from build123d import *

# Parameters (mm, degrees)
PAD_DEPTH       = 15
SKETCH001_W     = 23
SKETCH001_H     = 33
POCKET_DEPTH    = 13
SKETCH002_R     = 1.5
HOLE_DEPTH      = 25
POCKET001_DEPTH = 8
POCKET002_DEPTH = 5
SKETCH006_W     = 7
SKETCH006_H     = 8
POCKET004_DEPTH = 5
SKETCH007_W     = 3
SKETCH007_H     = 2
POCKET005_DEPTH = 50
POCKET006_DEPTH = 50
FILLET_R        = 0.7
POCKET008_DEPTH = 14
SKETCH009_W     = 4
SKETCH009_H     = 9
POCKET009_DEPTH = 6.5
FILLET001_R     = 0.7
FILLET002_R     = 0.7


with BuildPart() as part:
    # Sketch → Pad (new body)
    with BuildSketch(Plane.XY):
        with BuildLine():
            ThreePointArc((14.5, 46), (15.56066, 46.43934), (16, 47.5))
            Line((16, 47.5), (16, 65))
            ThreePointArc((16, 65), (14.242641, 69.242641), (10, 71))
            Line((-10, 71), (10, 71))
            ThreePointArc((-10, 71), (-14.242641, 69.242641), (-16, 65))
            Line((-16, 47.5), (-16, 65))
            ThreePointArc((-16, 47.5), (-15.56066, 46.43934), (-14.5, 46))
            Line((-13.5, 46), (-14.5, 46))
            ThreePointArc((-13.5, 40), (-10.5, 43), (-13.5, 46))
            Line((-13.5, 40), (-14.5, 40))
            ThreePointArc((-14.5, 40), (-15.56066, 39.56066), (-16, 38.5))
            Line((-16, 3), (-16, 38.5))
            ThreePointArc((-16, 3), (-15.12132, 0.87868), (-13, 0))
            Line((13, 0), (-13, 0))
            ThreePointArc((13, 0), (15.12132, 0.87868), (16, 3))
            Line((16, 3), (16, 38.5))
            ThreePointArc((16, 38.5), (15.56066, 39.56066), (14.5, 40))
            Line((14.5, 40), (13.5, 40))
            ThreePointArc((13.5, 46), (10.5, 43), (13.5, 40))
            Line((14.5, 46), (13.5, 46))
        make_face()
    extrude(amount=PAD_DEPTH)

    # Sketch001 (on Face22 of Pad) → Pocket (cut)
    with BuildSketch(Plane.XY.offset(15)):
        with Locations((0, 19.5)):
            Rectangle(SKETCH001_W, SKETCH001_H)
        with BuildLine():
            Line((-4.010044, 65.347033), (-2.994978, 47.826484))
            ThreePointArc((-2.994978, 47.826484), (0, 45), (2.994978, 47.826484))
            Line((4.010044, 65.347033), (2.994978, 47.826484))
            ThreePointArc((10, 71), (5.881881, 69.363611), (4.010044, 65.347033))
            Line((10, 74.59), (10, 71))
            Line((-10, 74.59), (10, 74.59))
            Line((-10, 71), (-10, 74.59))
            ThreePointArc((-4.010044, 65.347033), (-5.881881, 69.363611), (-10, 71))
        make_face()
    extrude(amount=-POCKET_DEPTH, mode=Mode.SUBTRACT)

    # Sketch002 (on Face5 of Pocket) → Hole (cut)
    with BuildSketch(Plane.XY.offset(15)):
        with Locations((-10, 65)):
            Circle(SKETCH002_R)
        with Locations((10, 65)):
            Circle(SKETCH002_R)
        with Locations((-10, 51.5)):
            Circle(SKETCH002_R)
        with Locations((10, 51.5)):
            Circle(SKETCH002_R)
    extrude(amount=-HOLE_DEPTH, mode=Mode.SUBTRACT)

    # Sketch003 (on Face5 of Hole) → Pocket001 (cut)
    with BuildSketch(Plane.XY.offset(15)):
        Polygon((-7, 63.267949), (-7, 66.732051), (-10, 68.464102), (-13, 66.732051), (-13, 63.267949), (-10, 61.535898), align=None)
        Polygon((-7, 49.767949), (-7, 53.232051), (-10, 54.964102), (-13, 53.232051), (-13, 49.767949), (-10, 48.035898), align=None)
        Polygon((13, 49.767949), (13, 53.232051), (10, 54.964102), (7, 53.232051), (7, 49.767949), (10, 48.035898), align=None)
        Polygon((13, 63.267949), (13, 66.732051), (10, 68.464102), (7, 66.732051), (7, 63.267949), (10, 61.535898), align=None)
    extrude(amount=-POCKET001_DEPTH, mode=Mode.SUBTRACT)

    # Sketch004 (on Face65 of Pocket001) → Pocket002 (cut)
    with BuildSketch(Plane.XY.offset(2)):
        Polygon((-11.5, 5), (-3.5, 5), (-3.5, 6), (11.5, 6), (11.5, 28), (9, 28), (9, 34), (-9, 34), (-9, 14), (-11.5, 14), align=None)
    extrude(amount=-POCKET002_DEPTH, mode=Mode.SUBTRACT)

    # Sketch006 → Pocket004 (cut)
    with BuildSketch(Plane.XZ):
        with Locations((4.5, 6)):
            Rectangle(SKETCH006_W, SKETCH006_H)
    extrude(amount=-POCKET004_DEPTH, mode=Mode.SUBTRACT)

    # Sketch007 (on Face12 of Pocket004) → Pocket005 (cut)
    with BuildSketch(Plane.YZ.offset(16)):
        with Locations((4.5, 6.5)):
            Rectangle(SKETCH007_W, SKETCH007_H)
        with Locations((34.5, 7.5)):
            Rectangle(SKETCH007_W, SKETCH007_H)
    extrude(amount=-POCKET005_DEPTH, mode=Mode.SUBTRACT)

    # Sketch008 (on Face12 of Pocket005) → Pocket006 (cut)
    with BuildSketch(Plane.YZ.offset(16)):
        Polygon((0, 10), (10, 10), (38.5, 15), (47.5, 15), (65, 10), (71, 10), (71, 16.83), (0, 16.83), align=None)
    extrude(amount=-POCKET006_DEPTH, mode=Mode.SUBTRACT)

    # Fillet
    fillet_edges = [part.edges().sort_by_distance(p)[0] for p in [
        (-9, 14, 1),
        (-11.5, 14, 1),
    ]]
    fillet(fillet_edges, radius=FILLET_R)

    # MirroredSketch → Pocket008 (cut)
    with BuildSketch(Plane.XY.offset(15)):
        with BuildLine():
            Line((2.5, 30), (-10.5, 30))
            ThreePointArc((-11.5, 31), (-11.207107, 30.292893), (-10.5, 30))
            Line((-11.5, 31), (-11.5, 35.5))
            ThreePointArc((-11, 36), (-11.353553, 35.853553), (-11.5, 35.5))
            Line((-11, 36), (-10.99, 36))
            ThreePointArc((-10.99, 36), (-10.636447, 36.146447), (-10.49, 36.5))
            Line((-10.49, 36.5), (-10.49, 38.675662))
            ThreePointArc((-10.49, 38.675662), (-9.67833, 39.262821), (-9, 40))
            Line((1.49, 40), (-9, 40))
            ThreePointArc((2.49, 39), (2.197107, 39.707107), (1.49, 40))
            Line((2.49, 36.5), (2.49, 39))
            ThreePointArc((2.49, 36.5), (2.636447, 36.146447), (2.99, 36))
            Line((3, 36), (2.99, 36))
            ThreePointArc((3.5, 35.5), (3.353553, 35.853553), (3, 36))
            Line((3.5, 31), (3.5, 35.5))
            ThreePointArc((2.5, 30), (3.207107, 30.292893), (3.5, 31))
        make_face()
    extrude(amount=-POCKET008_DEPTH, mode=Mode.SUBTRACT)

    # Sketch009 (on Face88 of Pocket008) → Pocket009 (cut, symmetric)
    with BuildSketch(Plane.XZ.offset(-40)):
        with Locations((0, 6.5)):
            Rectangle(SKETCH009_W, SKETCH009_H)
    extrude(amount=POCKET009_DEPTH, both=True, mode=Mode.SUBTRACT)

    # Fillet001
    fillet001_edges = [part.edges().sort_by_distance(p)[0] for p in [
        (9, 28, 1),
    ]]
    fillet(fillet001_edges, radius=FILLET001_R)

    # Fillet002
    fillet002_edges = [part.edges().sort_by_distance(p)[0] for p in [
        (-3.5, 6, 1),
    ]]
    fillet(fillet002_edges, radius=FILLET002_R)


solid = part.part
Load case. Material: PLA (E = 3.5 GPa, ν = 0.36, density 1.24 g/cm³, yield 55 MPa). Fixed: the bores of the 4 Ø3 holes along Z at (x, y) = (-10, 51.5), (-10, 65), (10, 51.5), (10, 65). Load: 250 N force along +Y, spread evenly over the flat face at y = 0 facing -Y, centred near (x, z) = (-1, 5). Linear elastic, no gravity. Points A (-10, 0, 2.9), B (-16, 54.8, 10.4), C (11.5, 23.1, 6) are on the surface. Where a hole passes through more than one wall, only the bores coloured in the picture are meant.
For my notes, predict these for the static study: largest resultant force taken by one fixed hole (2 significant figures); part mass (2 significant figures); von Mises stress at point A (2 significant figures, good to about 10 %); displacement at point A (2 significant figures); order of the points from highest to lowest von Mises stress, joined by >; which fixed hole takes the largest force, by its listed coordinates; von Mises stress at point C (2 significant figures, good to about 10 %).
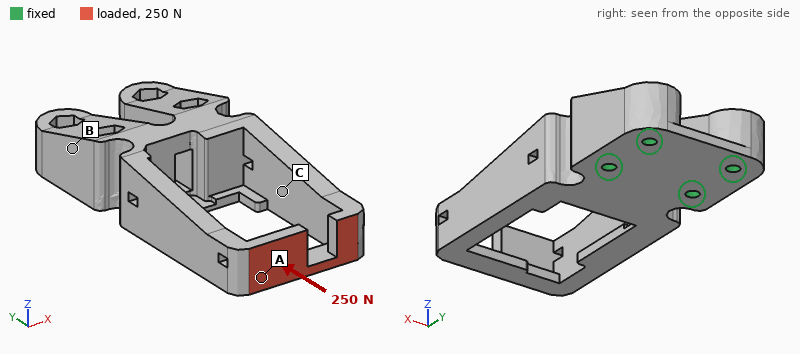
120 N
18 g
9.1 MPa
0.16 mm
A > C > B
(-10, 51.5)
5.7 MPa
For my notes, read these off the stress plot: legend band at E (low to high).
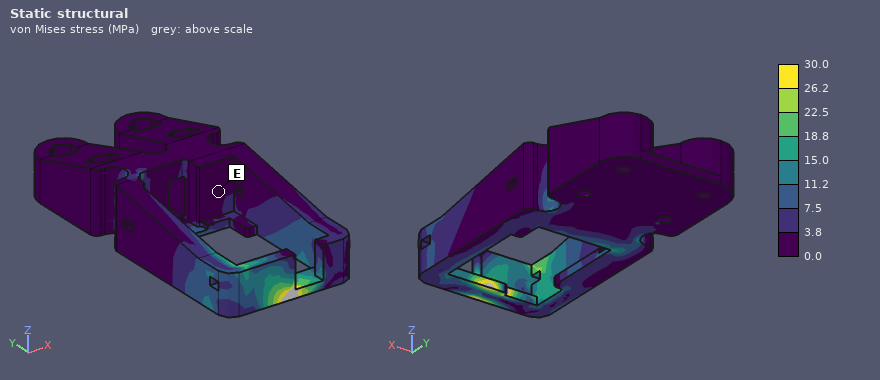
0.0 to 3.8 MPa
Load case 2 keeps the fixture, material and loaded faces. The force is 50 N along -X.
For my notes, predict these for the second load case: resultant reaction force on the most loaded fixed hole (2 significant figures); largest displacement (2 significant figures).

110 N
0.86 mm
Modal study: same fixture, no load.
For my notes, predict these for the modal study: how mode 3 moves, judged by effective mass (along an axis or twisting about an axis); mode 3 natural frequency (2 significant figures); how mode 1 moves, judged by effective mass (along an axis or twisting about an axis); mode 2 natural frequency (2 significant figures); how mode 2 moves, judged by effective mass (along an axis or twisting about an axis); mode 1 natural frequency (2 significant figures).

twisting about Y
1800 Hz
along X
1100 Hz
along Z
840 Hz
